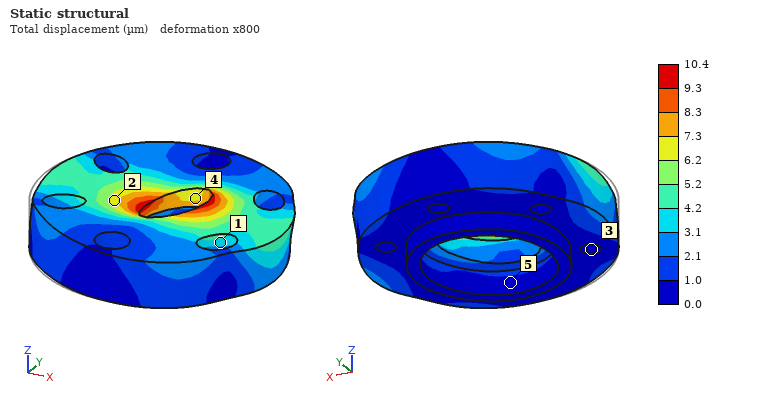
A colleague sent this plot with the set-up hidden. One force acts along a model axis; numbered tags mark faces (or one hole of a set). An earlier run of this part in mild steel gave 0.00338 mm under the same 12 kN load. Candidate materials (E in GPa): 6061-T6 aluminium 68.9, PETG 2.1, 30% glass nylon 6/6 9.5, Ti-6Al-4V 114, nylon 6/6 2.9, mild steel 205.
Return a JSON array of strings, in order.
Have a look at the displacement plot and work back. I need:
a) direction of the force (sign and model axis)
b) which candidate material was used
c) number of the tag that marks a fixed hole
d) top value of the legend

["+X", "6061-T6 aluminium", "3", "10.4 µm"]
